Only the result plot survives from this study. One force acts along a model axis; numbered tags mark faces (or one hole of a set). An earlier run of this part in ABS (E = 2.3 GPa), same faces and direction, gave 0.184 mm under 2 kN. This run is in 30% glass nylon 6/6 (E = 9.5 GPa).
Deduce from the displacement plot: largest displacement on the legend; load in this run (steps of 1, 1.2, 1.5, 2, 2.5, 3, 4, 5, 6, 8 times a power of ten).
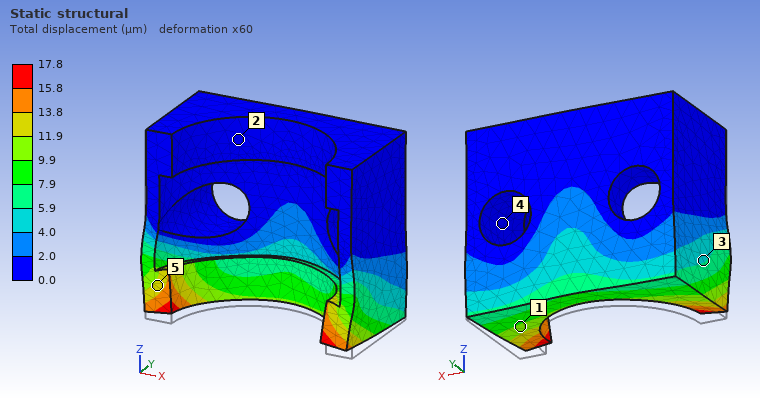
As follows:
17.8 µm
800 N
